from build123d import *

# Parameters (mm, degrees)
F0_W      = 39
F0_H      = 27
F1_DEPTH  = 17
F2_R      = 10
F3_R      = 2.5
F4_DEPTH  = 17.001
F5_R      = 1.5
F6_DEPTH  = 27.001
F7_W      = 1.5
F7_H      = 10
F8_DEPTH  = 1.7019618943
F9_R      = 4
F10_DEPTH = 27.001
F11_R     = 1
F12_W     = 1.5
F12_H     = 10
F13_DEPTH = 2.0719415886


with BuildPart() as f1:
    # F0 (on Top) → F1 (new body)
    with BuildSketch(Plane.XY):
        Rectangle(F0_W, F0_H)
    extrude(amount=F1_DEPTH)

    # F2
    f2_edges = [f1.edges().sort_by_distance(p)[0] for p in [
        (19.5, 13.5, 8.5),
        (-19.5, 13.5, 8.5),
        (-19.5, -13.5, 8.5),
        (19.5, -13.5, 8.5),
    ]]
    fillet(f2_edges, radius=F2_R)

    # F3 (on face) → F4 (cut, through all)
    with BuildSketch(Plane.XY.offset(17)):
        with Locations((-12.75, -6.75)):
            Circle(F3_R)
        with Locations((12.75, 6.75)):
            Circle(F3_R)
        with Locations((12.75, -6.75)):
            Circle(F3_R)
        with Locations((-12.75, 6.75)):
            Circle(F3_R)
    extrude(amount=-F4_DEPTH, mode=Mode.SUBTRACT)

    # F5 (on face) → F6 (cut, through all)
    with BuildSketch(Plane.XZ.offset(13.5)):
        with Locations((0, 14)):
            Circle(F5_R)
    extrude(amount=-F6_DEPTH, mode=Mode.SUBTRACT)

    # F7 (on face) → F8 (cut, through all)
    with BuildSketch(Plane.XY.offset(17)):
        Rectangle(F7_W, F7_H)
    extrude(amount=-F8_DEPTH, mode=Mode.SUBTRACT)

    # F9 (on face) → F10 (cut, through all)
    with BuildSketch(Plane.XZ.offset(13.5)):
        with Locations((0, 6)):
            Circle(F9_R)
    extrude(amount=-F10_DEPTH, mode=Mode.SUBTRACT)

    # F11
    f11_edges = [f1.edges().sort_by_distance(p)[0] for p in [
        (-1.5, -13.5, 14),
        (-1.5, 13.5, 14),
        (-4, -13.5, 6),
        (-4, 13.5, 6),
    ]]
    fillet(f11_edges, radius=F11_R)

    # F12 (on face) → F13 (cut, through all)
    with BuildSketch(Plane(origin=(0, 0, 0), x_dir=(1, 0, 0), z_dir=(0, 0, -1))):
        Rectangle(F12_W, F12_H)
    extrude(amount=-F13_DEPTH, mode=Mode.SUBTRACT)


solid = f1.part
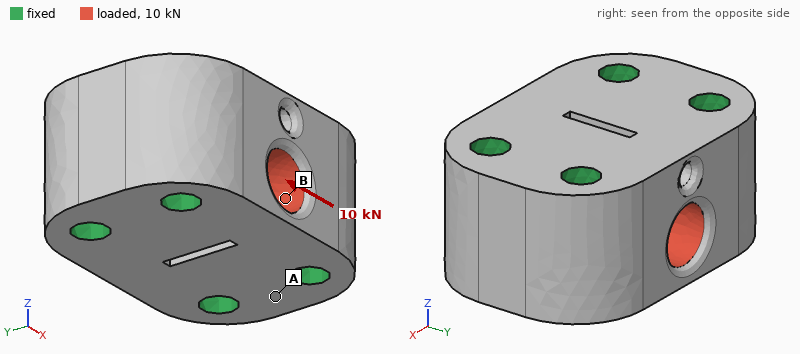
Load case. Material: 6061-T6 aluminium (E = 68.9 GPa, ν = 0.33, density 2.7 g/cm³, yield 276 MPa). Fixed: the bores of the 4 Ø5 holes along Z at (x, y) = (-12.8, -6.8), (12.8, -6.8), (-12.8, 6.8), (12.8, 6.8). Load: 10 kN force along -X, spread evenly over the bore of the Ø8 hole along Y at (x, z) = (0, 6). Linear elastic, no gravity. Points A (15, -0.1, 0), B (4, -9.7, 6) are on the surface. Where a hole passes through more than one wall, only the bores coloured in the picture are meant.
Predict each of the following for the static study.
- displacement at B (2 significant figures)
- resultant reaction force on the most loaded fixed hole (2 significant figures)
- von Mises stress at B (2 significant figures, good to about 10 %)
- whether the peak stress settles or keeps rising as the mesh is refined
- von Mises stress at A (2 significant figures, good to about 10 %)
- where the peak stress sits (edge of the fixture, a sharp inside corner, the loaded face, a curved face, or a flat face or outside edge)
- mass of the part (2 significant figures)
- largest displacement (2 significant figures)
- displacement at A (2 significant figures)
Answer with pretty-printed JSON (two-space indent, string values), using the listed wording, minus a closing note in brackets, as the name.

{
  "displacement at B": "1.9 µm",
  "resultant reaction force on the most loaded fixed hole": "2.5 kN",
  "von Mises stress at B": "15 MPa",
  "whether the peak stress settles or keeps rising as the mesh is refined": "keeps rising",
  "von Mises stress at A": "4.7 MPa",
  "where the peak stress sits": "edge of the fixture",
  "mass of the part": "36 g",
  "largest displacement": "2.9 µm",
  "displacement at A": "0.58 µm"
}
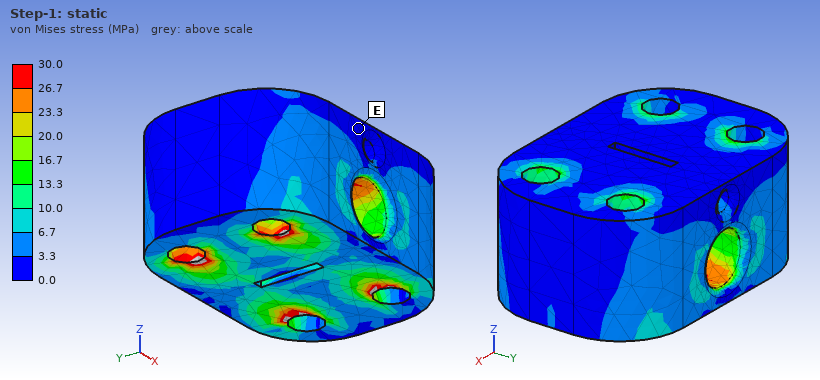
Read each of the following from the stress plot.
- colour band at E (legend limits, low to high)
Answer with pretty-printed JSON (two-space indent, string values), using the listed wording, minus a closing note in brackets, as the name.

{
  "colour band at E": "0.0 to 3.3 MPa"
}
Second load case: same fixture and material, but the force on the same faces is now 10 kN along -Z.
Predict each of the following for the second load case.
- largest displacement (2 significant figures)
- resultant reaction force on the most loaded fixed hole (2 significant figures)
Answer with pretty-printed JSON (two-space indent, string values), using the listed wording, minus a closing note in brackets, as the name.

{
  "largest displacement": "12 µm",
  "resultant reaction force on the most loaded fixed hole": "2.5 kN"
}
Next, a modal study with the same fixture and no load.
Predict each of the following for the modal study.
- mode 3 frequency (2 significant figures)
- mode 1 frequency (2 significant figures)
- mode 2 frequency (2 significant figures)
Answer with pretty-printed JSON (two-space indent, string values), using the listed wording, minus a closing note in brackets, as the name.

{
  "mode 3 frequency": "68 kHz",
  "mode 1 frequency": "64 kHz",
  "mode 2 frequency": "65 kHz"
}
